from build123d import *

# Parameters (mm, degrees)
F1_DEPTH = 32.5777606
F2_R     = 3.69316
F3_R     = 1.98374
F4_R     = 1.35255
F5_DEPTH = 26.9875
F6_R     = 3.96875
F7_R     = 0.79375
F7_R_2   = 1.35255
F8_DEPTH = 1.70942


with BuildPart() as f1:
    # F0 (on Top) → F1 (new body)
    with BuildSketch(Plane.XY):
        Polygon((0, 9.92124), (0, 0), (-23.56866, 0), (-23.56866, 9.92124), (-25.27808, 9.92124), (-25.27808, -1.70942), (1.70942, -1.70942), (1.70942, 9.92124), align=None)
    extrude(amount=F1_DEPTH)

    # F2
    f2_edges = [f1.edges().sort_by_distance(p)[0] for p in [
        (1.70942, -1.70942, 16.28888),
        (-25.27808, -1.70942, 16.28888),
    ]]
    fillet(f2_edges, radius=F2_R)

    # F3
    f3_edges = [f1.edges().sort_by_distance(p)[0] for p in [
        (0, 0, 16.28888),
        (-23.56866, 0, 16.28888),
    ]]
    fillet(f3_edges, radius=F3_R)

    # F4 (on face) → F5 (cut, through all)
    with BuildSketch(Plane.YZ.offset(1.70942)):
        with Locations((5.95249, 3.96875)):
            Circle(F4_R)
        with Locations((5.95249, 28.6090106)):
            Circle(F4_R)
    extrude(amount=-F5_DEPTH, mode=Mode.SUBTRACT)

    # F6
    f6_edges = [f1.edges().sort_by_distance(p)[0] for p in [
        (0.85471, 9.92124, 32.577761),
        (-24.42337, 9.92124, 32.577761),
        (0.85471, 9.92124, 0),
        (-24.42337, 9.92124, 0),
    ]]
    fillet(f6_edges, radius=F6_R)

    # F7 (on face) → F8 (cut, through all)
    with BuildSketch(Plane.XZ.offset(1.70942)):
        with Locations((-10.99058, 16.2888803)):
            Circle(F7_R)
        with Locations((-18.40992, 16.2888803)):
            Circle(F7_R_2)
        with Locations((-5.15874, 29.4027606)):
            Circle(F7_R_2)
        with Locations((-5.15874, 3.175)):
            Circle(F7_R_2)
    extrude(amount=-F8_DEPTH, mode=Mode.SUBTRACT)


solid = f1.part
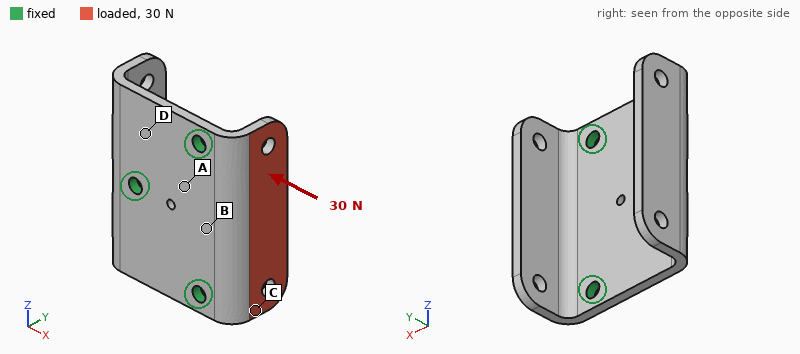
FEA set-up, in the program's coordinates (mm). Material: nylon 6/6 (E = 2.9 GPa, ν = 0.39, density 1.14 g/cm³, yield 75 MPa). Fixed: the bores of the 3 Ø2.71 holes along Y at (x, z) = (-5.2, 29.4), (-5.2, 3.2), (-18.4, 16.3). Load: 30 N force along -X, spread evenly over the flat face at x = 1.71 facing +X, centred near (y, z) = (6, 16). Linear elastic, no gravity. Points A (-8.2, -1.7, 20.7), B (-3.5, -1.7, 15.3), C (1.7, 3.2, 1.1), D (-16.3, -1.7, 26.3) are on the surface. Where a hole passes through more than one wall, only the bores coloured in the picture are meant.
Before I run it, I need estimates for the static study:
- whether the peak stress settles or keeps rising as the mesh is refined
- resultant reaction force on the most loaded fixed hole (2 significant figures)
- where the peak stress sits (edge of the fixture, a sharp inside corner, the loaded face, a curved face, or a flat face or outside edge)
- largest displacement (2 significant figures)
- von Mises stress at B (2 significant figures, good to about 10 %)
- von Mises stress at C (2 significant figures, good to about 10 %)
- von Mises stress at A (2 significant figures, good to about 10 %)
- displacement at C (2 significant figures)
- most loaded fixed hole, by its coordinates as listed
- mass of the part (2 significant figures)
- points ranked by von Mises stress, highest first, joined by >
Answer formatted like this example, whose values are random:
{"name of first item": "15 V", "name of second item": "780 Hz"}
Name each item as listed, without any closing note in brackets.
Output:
{"whether the peak stress settles or keeps rising as the mesh is refined": "keeps rising", "resultant reaction force on the most loaded fixed hole": "12 N", "where the peak stress sits": "edge of the fixture", "largest displacement": "0.41 mm", "von Mises stress at B": "7.5 MPa", "von Mises stress at C": "5.1 MPa", "von Mises stress at A": "3.0 MPa", "displacement at C": "0.16 mm", "most loaded fixed hole, by its coordinates as listed": "(-18.4, 16.3)", "mass of the part": "2.7 g", "points ranked by von Mises stress, highest first, joined by >": "B > C > A > D"}
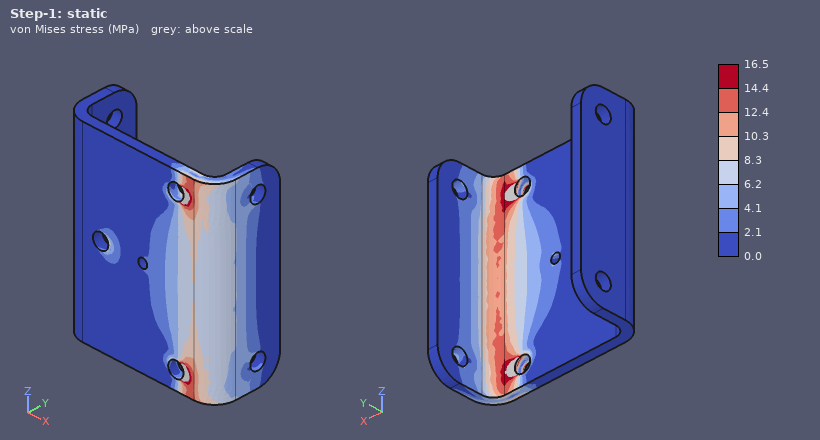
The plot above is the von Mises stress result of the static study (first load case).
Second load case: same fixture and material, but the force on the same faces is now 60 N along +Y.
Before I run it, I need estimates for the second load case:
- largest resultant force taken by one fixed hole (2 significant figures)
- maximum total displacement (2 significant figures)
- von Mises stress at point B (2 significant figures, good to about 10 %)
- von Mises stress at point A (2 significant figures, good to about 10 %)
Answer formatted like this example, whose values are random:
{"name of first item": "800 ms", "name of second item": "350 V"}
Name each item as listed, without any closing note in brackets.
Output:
{"largest resultant force taken by one fixed hole": "35 N", "maximum total displacement": "0.46 mm", "von Mises stress at point B": "7.1 MPa", "von Mises stress at point A": "4.3 MPa"}
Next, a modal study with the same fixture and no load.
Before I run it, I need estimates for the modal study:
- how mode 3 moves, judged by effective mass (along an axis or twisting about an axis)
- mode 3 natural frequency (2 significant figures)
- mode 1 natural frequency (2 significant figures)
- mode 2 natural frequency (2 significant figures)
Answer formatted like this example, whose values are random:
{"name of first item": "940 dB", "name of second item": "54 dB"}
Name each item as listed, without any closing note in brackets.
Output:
{"how mode 3 moves, judged by effective mass": "along X", "mode 3 natural frequency": "2300 Hz", "mode 1 natural frequency": "1700 Hz", "mode 2 natural frequency": "2100 Hz"}
